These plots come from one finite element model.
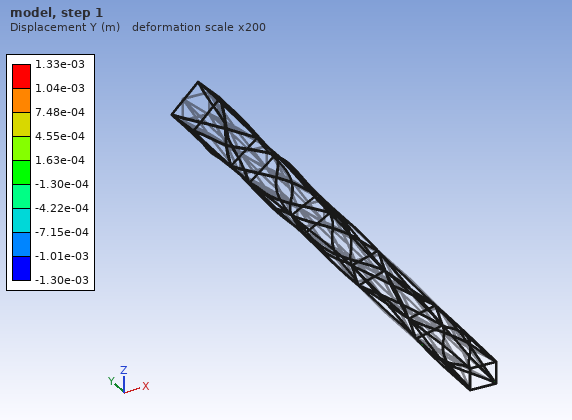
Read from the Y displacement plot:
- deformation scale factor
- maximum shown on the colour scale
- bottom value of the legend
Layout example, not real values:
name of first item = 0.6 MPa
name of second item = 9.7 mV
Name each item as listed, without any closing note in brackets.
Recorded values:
deformation scale factor = 200
maximum shown on the colour scale = 1.33e-03 m
bottom value of the legend = -1.30e-03 m
